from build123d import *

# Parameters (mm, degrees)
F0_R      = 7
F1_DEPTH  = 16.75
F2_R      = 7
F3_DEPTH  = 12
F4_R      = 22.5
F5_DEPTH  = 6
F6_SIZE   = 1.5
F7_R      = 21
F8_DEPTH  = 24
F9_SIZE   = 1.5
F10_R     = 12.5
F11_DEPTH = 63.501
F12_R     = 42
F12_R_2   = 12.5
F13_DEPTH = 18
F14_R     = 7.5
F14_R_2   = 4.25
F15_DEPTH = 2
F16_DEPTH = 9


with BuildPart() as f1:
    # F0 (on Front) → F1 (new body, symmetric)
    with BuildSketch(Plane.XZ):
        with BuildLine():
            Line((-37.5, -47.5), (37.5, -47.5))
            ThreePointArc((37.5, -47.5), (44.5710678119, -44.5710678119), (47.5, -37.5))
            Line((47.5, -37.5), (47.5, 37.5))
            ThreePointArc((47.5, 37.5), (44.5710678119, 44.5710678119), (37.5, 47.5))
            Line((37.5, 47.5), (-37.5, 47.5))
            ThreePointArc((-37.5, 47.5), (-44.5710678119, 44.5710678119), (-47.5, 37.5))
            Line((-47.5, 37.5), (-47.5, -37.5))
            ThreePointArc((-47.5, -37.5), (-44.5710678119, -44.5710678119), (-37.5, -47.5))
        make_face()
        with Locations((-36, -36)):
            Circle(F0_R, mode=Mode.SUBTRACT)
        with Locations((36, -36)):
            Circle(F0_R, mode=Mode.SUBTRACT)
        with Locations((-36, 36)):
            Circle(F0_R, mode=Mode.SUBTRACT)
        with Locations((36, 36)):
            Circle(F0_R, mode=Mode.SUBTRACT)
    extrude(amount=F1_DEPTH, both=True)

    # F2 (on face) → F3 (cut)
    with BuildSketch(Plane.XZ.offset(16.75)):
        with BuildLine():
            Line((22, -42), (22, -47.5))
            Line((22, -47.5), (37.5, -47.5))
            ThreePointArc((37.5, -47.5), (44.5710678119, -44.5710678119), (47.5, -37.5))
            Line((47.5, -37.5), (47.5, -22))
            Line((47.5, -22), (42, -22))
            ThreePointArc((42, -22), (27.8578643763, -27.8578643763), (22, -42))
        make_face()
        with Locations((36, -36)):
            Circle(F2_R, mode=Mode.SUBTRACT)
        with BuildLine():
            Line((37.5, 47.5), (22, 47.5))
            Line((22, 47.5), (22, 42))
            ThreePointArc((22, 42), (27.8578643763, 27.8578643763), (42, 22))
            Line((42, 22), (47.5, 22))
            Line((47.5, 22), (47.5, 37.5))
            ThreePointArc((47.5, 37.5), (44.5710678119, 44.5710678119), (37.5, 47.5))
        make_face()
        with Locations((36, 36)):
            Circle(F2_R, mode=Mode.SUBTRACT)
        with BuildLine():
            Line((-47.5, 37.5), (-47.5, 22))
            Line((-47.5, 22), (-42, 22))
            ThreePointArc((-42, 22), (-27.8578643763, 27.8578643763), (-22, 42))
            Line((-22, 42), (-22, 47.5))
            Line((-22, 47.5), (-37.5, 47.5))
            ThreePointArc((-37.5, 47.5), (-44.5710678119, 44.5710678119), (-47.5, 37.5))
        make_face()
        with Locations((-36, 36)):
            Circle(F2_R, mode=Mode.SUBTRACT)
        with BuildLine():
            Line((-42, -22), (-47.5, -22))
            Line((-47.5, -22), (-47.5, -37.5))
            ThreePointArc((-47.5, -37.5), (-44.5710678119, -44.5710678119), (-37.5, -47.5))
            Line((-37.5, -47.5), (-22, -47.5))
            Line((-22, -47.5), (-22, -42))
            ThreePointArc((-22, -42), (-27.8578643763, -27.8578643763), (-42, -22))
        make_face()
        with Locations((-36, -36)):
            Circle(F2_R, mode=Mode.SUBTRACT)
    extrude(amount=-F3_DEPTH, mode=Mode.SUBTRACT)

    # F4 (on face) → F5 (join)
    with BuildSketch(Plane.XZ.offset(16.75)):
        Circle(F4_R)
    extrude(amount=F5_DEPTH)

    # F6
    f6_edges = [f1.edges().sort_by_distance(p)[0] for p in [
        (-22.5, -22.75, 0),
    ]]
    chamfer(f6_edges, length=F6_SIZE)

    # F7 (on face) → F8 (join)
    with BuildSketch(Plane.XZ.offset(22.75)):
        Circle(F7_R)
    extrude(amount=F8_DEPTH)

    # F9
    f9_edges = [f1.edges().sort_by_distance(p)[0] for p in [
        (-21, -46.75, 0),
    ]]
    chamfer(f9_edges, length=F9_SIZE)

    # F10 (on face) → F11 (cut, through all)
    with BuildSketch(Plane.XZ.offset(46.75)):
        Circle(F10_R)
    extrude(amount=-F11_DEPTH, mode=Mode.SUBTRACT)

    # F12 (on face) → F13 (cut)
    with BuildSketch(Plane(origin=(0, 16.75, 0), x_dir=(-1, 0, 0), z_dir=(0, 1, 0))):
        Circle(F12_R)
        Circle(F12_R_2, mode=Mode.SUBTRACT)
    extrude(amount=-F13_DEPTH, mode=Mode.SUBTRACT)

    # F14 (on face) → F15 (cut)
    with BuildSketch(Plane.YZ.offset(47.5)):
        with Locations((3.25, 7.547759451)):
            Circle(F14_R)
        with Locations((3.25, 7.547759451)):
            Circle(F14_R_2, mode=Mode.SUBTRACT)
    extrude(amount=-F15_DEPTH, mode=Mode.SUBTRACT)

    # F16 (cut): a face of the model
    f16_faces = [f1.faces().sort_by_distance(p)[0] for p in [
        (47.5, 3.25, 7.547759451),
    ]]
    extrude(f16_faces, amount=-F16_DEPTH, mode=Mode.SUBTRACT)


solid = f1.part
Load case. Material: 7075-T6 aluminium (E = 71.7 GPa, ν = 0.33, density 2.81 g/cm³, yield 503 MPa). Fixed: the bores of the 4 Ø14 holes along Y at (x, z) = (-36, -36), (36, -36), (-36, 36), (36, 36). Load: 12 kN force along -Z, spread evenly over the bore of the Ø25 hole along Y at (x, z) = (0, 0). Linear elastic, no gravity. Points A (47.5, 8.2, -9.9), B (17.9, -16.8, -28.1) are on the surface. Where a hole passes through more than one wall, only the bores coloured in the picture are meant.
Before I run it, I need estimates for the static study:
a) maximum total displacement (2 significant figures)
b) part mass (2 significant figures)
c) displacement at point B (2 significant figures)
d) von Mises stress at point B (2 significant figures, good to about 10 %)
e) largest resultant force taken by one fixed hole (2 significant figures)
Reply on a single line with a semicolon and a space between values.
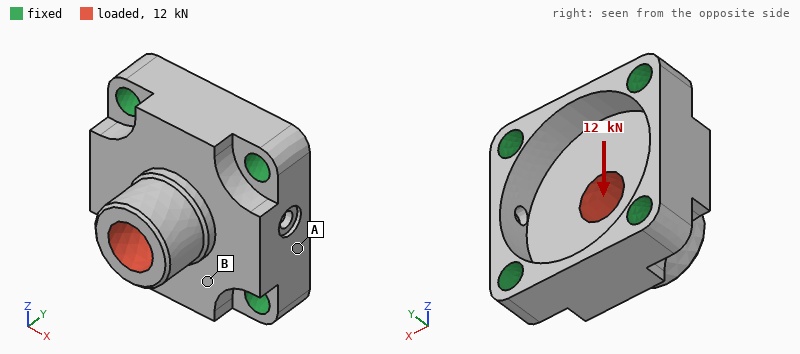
28 µm; 510 g; 5.9 µm; 6.4 MPa; 3.9 kN
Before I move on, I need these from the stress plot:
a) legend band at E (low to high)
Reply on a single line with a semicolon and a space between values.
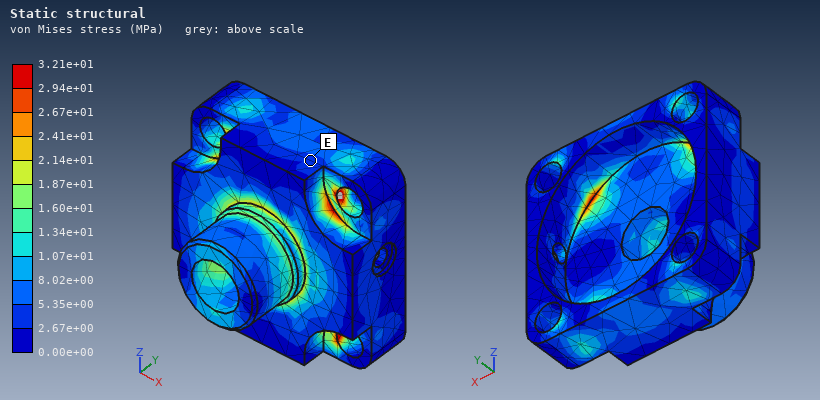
2.67e+00 to 5.35e+00 MPa
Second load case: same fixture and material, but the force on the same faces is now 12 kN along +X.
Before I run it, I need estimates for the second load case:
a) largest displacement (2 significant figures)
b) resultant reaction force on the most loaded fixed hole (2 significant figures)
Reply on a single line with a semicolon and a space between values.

28 µm; 3.9 kN
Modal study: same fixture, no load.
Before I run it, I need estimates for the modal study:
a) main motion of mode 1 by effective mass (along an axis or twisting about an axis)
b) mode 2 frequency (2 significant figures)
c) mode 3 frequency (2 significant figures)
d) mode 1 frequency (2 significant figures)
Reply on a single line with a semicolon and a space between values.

along Y; 10 kHz; 10 kHz; 9200 Hz
